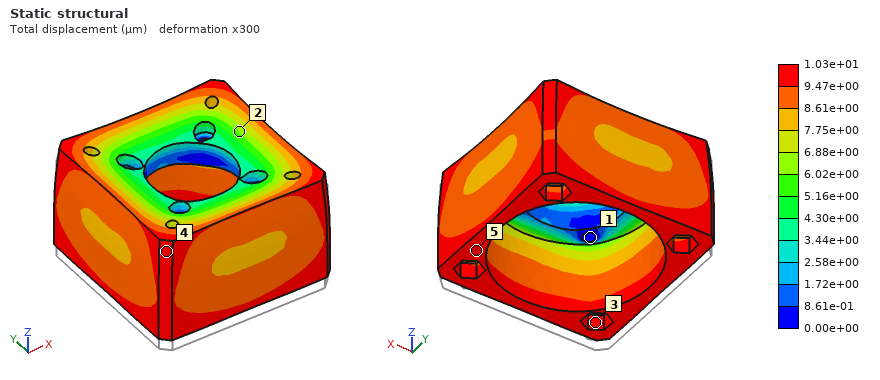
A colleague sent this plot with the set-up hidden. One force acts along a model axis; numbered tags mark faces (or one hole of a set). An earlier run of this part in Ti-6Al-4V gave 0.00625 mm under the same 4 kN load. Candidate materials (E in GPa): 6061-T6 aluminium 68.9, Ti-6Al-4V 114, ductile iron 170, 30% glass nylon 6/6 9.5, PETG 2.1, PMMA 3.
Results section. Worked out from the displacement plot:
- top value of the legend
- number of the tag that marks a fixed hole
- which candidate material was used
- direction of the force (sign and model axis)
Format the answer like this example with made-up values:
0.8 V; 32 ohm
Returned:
1.03e+01 µm; 1; 6061-T6 aluminium; +Z
